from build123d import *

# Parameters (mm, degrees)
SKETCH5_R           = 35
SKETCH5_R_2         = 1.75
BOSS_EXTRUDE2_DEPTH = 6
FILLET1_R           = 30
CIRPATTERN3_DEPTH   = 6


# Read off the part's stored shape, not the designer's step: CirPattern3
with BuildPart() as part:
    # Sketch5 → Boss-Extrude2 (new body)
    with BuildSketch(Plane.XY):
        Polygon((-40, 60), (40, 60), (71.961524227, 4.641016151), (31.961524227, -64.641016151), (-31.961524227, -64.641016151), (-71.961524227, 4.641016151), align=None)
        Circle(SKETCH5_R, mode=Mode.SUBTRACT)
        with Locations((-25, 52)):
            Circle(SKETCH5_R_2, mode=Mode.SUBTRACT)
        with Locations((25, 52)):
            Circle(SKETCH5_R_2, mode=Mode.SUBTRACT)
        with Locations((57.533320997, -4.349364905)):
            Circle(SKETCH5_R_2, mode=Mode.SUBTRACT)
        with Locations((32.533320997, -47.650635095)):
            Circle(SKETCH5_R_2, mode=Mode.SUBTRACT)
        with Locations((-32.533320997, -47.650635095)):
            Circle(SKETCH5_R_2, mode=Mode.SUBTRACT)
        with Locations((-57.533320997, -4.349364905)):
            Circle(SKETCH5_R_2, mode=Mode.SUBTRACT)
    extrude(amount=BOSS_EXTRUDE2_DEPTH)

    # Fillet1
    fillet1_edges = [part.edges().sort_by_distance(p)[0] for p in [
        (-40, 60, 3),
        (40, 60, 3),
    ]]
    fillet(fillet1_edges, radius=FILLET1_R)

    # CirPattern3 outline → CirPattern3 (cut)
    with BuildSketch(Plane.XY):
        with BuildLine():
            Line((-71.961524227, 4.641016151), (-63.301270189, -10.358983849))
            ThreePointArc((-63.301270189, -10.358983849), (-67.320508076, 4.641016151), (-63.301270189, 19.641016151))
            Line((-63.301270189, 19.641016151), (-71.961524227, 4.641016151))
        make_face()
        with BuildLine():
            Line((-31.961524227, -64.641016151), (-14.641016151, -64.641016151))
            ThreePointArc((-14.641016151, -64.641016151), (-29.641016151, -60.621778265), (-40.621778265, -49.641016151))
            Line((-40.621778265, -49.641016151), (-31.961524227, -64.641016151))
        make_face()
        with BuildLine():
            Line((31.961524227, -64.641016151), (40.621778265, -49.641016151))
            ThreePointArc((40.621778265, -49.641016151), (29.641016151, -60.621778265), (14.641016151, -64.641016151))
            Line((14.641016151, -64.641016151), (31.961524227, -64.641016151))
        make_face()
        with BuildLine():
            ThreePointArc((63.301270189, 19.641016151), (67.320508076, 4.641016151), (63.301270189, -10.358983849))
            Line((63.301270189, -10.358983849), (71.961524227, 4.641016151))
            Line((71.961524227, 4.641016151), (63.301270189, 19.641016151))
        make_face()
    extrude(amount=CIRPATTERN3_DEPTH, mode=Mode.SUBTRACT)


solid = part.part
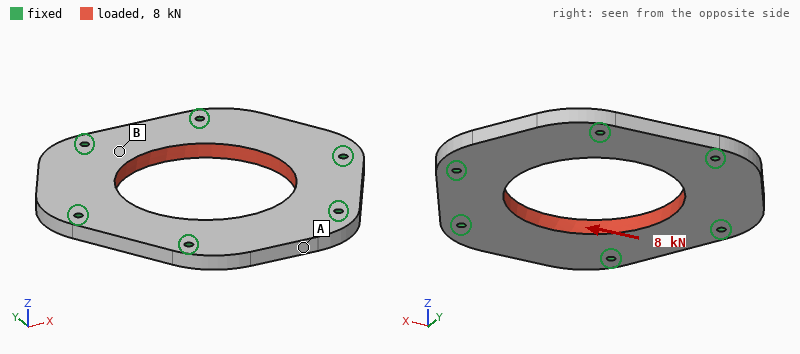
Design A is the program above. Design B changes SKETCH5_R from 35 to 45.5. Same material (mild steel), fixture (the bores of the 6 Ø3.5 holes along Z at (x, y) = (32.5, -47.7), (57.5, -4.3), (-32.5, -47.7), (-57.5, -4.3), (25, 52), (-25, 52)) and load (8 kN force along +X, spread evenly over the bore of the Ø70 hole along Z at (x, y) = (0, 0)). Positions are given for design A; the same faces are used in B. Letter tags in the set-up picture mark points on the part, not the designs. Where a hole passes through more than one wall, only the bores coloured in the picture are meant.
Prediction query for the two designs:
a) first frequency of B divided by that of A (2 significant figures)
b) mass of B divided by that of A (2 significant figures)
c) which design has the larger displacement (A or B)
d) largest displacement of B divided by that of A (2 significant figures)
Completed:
1.0
0.71
B
1.3
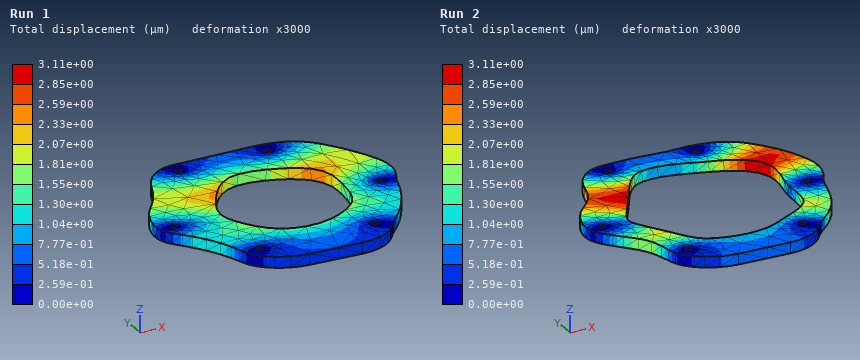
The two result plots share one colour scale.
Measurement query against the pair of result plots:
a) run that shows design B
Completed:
Run 2
